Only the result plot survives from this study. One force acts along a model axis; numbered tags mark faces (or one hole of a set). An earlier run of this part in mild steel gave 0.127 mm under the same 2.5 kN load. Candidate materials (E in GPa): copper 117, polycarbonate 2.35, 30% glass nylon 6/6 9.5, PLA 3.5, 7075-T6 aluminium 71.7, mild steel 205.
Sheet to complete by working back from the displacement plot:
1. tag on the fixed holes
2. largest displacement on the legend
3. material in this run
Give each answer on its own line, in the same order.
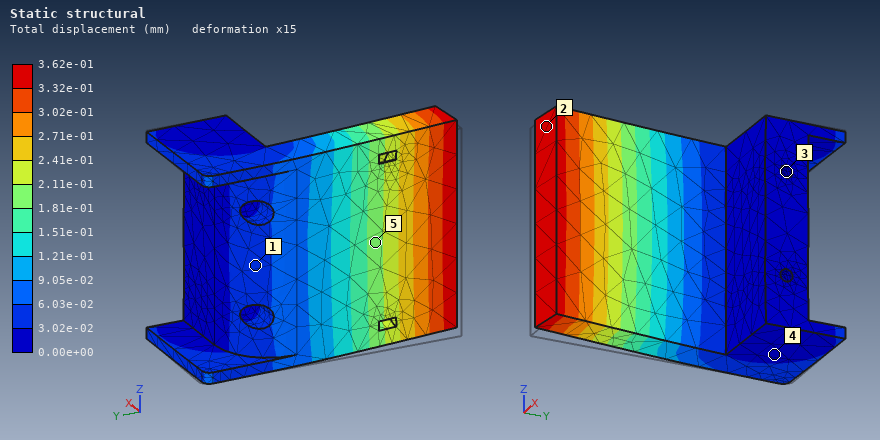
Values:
3
3.62e-01 mm
7075-T6 aluminium
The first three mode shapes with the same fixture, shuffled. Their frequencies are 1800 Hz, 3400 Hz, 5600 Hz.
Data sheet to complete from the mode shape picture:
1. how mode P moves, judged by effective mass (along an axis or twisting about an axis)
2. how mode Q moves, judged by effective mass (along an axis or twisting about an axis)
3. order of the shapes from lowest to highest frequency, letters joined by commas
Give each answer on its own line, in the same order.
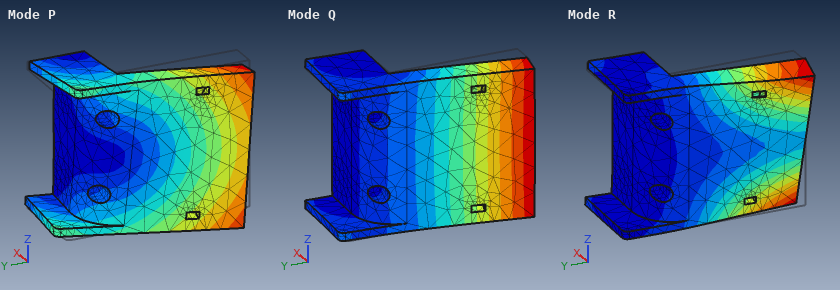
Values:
along Z
along X
Q, P, R
